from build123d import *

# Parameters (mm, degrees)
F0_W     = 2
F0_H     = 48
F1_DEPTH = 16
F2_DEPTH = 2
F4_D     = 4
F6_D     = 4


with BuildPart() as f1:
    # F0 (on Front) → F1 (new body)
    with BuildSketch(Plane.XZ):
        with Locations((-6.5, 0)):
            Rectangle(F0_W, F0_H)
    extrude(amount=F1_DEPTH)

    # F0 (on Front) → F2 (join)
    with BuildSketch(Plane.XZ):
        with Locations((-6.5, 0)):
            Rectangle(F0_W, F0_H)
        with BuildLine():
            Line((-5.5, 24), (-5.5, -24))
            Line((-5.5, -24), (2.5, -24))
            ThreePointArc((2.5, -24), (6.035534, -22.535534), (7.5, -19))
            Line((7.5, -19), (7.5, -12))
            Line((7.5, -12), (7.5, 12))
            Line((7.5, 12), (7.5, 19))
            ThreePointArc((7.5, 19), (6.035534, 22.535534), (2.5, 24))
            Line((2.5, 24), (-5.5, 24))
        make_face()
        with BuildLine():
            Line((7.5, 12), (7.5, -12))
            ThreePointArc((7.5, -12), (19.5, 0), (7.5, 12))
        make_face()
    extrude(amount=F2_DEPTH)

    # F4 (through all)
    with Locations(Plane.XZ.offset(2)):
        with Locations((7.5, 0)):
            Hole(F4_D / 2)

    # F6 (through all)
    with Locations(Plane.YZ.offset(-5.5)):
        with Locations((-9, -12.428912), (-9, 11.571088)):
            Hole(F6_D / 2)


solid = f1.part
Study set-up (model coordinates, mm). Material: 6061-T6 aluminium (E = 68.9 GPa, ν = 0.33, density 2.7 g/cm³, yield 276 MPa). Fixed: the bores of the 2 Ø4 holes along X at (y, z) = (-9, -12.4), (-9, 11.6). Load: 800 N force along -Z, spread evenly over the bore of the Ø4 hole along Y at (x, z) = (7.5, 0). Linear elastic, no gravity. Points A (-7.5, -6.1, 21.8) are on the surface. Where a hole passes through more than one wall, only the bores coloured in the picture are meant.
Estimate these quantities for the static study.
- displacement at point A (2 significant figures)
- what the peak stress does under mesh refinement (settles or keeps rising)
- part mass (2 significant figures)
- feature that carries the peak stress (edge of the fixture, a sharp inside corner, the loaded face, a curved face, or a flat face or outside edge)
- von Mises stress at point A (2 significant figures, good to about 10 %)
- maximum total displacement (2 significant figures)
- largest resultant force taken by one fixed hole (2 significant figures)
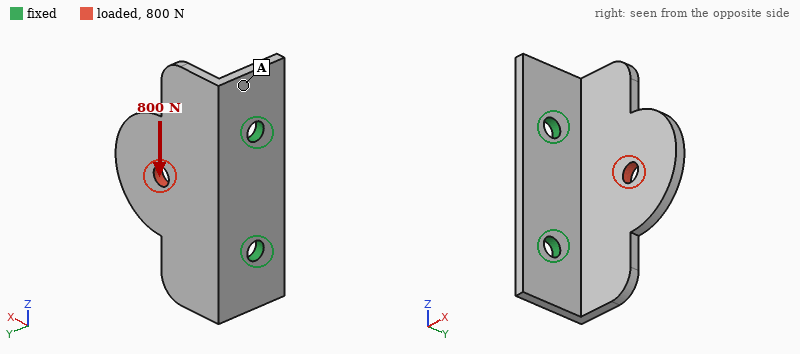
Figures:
0.043 mm
keeps rising
8.5 g
edge of the fixture
38 MPa
0.14 mm
620 N
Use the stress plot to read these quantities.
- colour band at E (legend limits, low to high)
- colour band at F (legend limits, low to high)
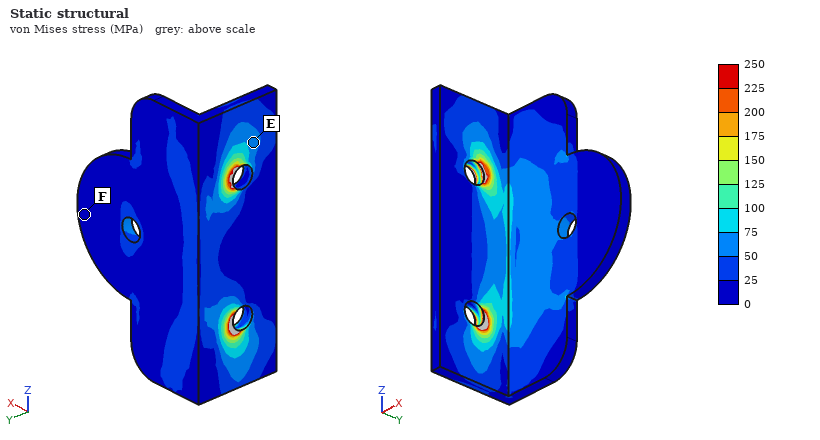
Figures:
50 to 75 MPa
0 to 25 MPa
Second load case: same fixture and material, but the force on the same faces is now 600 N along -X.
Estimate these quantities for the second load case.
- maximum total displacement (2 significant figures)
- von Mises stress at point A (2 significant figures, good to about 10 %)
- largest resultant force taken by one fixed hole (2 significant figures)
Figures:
0.23 mm
40 MPa
310 N
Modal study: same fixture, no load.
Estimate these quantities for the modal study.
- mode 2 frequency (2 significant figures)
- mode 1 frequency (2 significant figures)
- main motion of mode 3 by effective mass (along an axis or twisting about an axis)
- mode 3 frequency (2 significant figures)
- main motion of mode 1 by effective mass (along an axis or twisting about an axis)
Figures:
5500 Hz
2500 Hz
along X
8300 Hz
along Y
